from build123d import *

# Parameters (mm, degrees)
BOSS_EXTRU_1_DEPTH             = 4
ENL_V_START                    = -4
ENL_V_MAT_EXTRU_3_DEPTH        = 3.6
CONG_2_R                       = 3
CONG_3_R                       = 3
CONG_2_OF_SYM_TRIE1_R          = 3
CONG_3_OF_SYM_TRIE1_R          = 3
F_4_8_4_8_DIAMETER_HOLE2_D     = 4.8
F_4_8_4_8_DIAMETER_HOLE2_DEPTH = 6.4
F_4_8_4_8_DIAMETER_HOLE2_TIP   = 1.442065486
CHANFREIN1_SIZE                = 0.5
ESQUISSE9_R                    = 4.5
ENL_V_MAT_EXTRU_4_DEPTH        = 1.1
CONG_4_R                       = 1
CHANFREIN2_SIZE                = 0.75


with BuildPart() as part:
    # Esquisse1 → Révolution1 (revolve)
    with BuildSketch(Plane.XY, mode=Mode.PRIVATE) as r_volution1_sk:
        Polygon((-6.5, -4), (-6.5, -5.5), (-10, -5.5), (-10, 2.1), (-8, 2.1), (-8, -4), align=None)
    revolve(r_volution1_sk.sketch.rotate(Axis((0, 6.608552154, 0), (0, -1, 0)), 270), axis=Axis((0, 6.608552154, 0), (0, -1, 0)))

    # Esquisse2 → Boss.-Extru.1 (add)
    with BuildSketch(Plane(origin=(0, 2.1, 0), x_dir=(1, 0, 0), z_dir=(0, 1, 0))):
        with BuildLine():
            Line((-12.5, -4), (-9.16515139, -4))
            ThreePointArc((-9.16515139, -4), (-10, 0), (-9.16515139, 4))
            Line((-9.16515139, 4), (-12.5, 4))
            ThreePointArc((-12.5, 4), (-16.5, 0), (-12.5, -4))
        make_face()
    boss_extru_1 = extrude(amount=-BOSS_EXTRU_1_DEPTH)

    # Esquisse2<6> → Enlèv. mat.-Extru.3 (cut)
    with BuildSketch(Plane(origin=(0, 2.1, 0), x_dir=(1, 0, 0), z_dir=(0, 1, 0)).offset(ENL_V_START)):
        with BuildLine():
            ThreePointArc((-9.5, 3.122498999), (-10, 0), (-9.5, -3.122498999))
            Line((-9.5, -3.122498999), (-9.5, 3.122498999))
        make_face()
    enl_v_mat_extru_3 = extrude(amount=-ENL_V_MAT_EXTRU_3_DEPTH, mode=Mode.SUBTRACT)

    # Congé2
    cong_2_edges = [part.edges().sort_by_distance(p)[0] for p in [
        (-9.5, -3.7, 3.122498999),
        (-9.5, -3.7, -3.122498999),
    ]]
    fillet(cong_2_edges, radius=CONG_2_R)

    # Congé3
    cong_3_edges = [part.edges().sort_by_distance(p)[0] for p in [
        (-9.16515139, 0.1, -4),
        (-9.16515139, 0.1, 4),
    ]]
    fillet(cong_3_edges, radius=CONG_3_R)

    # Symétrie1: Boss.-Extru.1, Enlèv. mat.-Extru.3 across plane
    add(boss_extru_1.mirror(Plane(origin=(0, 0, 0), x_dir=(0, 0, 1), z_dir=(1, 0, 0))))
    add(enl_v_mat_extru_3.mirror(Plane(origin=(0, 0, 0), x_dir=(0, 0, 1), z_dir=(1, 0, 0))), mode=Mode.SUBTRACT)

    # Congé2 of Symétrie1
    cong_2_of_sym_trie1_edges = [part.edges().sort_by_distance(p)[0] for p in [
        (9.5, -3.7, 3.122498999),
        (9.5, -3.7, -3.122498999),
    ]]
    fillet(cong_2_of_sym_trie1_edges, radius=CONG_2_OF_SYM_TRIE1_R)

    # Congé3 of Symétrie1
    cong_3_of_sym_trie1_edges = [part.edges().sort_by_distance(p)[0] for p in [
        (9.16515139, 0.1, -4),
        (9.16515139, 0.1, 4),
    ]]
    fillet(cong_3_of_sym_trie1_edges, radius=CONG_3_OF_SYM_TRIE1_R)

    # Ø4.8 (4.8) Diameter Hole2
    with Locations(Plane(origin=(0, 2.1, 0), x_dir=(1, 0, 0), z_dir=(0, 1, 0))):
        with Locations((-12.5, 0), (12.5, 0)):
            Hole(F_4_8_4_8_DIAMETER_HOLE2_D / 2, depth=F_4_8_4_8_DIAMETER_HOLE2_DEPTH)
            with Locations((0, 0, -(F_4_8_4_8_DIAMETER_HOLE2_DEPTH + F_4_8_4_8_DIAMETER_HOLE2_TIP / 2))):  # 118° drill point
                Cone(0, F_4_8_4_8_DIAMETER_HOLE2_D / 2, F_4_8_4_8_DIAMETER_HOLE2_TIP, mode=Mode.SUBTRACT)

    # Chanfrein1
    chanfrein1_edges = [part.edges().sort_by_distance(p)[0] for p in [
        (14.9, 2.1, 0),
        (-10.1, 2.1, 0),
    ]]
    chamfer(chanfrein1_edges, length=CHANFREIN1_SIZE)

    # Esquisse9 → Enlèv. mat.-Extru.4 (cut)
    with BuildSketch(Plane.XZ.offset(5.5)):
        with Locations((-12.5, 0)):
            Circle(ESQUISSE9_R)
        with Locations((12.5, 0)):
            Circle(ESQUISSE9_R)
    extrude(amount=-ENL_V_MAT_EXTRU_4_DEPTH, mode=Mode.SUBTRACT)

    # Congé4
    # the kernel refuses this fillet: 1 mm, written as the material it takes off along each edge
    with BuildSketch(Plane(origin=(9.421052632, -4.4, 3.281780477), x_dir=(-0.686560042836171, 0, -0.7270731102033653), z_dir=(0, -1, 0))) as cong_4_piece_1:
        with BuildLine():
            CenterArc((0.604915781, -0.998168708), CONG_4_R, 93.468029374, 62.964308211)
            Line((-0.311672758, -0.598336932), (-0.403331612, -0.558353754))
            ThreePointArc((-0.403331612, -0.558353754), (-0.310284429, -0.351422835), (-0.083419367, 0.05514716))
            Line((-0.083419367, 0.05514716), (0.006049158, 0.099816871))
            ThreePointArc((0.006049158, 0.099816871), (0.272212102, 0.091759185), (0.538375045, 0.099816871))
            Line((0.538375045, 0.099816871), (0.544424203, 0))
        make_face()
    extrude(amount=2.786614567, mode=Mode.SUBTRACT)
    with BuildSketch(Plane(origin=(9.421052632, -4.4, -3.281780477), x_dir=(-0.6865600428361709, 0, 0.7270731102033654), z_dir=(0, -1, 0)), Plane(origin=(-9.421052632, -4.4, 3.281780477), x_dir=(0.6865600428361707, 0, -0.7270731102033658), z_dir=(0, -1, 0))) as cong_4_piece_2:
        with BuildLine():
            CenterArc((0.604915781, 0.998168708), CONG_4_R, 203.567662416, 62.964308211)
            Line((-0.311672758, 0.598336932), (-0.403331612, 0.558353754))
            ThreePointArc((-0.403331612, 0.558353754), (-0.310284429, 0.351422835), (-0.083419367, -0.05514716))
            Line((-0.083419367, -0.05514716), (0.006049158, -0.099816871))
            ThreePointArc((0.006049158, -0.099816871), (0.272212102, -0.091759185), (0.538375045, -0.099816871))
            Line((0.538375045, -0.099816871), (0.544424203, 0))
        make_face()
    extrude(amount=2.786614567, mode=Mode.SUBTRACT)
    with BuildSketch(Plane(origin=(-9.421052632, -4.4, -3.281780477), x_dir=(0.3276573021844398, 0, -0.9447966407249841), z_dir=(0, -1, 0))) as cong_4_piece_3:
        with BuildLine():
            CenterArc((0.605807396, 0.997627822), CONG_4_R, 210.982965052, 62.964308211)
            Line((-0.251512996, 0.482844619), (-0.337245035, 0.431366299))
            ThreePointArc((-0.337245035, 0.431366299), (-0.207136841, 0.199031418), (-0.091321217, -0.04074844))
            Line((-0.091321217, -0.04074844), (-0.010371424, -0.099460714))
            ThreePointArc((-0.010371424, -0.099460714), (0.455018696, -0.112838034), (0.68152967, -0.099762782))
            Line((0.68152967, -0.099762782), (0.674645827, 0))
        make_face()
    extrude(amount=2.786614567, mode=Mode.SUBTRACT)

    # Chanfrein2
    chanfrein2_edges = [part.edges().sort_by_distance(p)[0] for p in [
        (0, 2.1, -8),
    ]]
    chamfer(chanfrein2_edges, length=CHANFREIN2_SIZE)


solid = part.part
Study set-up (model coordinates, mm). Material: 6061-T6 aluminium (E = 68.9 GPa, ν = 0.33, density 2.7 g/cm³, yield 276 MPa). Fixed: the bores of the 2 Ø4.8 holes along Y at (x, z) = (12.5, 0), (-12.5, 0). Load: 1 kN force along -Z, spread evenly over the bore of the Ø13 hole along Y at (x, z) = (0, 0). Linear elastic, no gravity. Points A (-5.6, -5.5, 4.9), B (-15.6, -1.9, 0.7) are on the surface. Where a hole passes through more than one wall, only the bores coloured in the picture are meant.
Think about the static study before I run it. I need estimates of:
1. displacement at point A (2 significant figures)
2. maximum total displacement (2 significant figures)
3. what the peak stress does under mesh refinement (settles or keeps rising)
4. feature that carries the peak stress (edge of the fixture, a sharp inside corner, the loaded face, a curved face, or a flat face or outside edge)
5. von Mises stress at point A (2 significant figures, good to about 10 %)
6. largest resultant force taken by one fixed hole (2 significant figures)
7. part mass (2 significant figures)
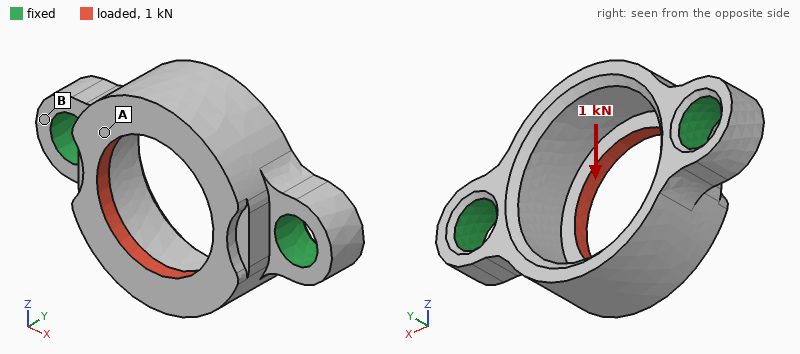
20 µm
33 µm
keeps rising
edge of the fixture
41 MPa
500 N
3.1 g
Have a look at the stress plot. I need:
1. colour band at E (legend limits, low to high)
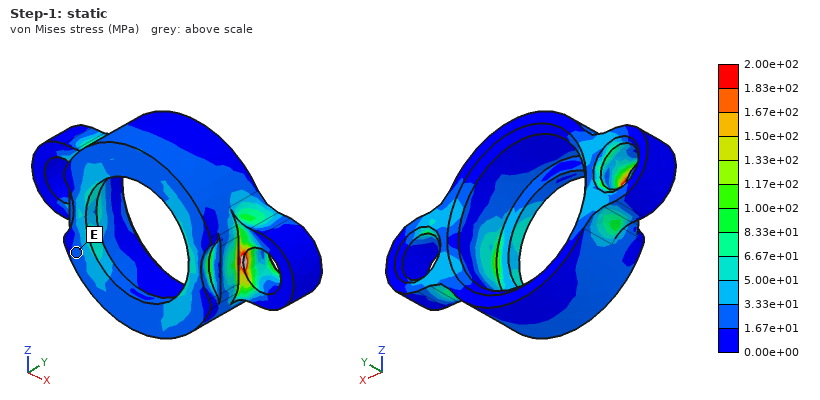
1.67e+01 to 3.33e+01 MPa
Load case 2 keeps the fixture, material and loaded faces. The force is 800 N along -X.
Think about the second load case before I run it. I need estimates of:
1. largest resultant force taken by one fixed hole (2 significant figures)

430 N
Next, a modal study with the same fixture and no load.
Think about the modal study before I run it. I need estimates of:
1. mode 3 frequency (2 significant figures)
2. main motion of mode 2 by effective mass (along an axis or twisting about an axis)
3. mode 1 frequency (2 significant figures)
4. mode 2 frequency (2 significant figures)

36 kHz
along Y
20 kHz
27 kHz
